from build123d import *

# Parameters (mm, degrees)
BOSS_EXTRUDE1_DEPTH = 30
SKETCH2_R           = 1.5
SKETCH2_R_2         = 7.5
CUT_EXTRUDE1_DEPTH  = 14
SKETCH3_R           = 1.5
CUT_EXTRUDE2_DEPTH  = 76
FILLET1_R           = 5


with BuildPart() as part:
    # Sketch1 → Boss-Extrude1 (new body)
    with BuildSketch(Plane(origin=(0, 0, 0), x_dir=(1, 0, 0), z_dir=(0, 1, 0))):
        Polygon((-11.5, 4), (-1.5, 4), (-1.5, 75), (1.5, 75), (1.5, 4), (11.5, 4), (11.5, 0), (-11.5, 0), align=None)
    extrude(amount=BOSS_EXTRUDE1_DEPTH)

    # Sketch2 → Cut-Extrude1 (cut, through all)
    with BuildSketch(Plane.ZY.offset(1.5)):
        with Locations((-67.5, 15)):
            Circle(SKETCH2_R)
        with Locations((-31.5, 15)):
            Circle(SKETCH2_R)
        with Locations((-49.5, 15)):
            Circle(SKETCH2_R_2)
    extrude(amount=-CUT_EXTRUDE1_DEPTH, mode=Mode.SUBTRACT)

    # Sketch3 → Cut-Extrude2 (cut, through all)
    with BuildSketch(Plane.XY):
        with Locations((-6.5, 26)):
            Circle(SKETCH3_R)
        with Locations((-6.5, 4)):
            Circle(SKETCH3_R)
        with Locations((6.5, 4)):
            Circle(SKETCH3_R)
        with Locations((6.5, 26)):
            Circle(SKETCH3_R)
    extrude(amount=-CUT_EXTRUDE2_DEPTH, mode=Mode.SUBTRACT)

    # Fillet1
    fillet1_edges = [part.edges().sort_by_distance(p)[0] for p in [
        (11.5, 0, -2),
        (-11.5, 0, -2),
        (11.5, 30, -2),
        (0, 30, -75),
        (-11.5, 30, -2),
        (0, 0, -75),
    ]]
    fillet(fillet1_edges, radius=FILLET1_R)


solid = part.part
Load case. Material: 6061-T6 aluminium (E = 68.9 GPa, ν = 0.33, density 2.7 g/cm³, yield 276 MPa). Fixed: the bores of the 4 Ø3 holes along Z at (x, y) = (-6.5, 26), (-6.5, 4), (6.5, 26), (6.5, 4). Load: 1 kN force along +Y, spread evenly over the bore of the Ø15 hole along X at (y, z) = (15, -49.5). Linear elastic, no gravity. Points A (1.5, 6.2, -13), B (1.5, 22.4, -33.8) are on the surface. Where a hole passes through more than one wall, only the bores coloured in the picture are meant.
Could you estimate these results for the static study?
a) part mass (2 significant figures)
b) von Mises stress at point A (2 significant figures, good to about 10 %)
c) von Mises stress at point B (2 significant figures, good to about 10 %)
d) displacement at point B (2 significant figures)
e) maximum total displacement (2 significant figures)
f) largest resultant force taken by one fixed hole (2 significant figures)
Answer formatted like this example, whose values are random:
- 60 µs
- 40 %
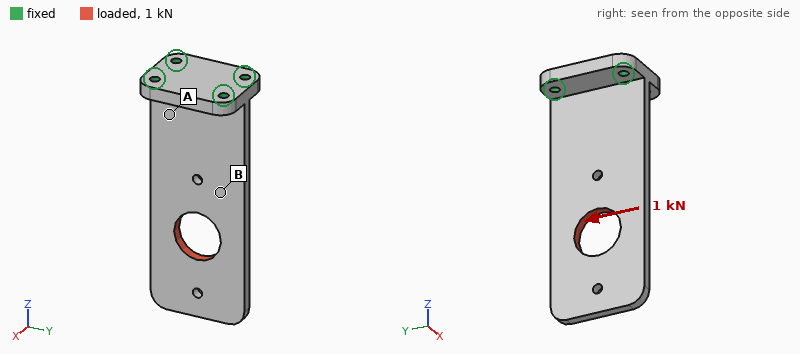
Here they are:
- 23 g
- 51 MPa
- 23 MPa
- 0.083 mm
- 0.24 mm
- 1.1 kN
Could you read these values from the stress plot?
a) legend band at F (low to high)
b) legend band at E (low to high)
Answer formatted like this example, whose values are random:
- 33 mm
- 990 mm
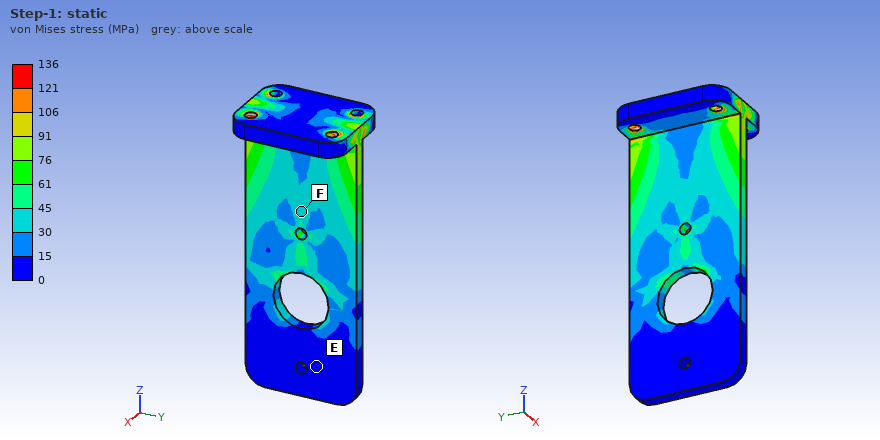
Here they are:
- 30 to 45 MPa
- 0 to 15 MPa
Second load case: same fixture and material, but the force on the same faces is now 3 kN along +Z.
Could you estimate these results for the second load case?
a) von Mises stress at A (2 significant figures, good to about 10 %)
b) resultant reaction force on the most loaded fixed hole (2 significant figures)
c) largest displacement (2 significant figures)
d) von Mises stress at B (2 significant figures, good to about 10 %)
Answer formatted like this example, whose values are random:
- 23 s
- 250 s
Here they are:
- 34 MPa
- 760 N
- 39 µm
- 36 MPa
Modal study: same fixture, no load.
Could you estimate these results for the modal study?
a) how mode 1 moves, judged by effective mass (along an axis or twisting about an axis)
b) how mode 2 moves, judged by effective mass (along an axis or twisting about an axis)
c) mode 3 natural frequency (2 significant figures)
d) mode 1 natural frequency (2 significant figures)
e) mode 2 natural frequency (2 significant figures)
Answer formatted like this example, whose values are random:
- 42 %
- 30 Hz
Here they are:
- along X
- twisting about Z
- 2800 Hz
- 500 Hz
- 2300 Hz
